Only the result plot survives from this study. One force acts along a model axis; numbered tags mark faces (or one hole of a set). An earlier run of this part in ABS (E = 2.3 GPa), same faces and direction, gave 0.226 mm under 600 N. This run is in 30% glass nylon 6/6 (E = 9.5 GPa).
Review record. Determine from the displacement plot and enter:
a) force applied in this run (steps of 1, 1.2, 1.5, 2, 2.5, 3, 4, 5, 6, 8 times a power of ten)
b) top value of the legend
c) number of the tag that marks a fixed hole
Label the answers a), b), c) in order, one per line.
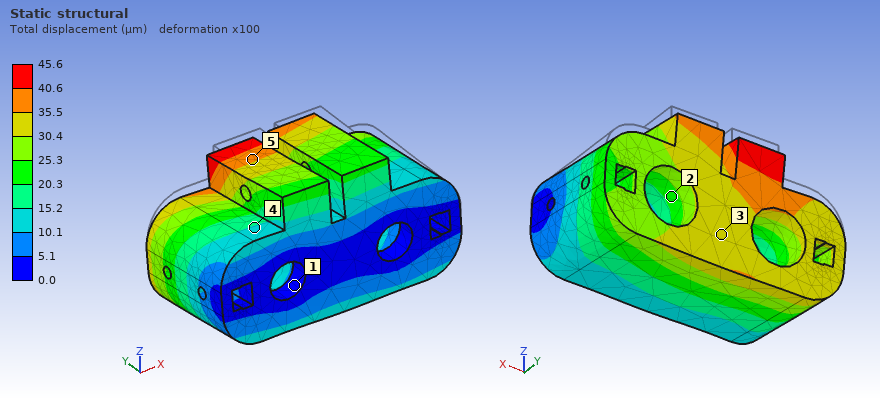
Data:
a) 500 N
b) 45.6 µm
c) 1
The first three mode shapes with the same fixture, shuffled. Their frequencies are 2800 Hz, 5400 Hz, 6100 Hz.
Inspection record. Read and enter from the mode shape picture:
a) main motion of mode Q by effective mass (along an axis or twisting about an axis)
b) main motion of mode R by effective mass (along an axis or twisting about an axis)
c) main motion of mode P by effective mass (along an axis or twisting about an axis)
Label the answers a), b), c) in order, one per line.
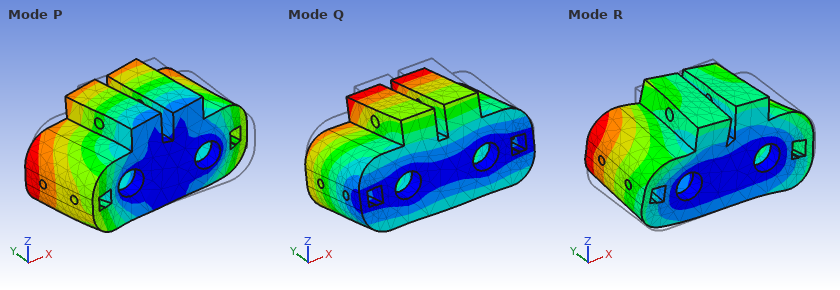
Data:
a) along Z
b) twisting about Y
c) along X
